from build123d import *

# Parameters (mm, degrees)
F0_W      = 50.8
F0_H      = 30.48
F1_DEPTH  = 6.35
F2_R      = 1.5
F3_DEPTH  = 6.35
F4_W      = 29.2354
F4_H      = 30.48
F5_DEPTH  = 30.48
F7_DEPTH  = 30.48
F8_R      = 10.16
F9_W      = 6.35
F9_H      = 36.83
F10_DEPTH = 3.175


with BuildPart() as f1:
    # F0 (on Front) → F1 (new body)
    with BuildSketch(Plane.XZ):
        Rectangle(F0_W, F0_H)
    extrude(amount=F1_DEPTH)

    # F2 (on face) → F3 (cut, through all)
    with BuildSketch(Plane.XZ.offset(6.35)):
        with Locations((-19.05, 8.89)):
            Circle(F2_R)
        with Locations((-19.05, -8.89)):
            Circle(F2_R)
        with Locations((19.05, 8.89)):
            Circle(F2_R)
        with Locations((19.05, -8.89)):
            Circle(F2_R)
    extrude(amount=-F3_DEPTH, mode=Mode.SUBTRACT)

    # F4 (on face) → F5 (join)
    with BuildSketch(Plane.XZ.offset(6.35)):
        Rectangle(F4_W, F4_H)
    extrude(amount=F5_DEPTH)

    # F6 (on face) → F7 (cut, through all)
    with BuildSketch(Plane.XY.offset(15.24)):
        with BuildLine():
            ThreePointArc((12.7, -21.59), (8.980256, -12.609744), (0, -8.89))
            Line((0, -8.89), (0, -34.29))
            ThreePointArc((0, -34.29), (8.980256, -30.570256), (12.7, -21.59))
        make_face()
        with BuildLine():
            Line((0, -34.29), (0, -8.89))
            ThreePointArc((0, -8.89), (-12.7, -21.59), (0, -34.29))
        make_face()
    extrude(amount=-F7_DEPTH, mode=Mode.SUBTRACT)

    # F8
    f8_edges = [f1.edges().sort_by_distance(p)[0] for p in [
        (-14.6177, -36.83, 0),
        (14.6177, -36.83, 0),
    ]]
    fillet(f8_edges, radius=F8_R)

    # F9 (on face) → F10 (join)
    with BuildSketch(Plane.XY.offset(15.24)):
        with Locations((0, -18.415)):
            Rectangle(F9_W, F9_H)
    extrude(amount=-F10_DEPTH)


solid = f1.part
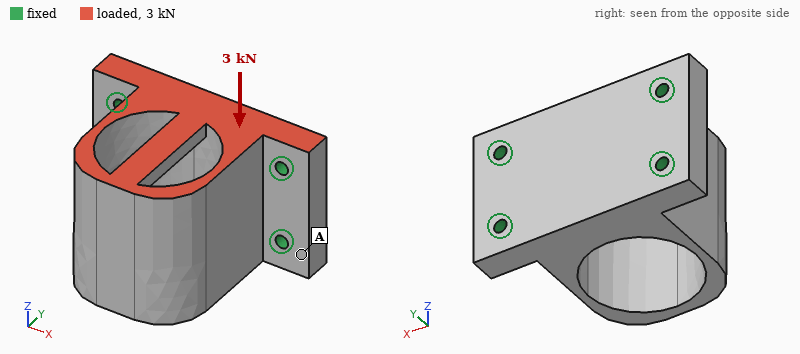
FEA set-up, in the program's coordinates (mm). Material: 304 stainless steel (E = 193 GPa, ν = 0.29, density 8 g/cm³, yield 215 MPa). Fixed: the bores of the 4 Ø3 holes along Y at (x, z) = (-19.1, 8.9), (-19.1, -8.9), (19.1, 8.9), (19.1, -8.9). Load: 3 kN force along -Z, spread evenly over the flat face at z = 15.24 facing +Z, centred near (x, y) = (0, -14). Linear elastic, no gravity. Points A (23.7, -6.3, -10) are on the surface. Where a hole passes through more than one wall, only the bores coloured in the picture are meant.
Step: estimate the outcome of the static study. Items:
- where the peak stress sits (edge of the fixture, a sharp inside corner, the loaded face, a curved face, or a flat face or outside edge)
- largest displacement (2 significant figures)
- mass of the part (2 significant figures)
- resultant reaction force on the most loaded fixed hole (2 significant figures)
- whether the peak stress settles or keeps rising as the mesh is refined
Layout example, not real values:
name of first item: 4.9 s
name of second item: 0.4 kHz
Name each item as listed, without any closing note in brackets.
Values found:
where the peak stress sits: edge of the fixture
largest displacement: 20 µm
mass of the part: 160 g
resultant reaction force on the most loaded fixed hole: 1.2 kN
whether the peak stress settles or keeps rising as the mesh is refined: keeps rising
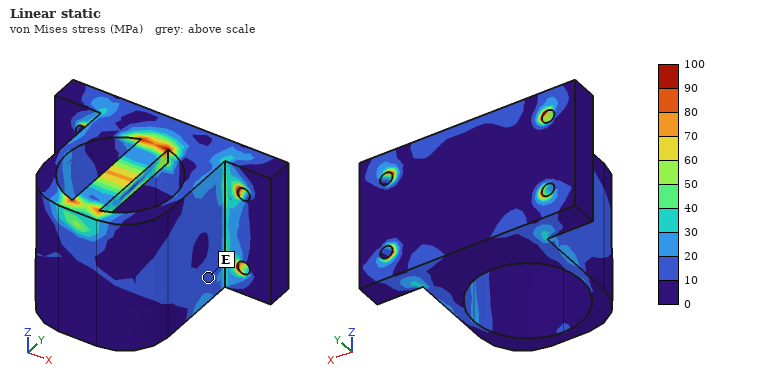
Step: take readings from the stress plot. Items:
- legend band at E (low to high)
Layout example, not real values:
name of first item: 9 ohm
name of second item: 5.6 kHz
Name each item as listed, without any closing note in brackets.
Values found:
legend band at E: 10 to 20 MPa
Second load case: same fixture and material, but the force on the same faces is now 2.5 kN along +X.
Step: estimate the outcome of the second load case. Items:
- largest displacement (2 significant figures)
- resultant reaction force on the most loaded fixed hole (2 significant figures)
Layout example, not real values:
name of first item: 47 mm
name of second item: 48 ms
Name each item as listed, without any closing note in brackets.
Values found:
largest displacement: 20 µm
resultant reaction force on the most loaded fixed hole: 1.1 kN
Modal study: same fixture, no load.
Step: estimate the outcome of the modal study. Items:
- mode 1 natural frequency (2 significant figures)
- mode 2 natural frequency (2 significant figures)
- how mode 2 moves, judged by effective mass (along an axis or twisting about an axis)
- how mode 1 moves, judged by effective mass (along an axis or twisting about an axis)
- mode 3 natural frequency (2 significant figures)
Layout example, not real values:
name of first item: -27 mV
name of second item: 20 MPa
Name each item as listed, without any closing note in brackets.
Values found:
mode 1 natural frequency: 5700 Hz
mode 2 natural frequency: 7800 Hz
how mode 2 moves, judged by effective mass: along Z
how mode 1 moves, judged by effective mass: along X
mode 3 natural frequency: 13 kHz
